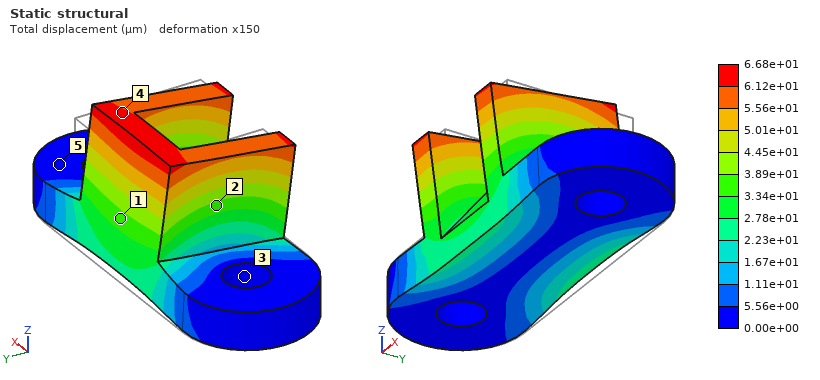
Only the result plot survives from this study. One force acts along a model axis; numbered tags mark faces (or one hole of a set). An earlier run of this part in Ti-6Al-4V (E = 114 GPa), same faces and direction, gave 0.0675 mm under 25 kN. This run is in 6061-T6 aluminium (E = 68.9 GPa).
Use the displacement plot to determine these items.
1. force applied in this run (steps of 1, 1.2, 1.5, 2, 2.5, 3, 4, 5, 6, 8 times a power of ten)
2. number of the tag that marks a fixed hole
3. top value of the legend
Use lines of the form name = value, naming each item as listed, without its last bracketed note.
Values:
force applied in this run = 15 kN
number of the tag that marks a fixed hole = 3
top value of the legend = 6.68e+01 µm
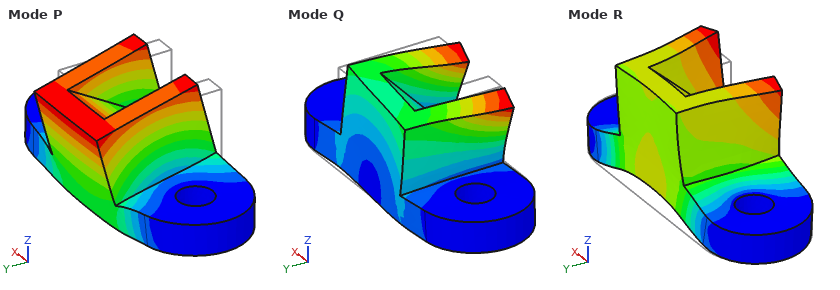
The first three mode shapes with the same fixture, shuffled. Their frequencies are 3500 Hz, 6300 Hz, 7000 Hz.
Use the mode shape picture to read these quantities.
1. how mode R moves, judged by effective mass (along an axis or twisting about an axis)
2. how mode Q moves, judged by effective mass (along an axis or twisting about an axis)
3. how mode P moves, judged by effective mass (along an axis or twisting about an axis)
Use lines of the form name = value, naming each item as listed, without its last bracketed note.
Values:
how mode R moves, judged by effective mass = along Z
how mode Q moves, judged by effective mass = along X
how mode P moves, judged by effective mass = along Y
